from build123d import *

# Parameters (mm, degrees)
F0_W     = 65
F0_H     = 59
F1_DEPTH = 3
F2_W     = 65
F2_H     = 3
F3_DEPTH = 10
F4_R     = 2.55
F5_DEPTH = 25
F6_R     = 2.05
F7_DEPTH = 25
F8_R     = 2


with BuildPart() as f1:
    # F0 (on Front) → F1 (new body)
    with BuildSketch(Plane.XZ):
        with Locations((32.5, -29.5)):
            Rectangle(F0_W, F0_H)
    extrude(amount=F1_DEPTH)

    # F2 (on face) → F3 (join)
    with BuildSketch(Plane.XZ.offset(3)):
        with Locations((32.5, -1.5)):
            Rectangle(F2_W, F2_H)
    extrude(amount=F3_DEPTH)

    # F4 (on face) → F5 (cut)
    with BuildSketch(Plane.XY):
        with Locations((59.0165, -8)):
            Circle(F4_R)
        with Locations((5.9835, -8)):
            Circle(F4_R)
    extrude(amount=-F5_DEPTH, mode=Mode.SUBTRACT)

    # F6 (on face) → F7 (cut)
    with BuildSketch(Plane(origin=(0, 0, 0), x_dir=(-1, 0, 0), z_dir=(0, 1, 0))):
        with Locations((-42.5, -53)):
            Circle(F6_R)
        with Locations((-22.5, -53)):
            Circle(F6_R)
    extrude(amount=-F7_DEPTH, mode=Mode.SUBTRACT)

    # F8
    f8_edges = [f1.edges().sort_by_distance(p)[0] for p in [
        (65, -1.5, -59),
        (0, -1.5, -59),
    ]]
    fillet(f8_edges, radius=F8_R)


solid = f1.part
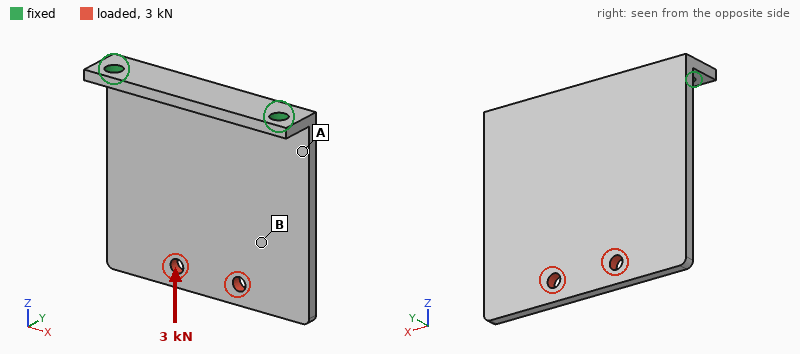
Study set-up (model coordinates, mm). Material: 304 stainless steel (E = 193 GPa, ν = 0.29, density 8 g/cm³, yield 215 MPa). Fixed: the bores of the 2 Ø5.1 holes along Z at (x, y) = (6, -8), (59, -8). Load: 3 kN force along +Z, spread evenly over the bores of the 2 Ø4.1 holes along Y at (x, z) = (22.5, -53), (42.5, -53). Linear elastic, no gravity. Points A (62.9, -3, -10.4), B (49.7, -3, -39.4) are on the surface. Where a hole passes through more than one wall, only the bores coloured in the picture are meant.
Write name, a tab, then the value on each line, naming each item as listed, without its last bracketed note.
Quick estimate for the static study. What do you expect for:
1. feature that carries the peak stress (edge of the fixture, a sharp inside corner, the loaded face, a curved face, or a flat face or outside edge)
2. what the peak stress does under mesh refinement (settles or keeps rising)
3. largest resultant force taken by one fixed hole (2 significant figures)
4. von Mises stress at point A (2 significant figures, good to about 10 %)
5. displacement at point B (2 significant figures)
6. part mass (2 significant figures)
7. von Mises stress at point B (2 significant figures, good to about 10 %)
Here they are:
feature that carries the peak stress	edge of the fixture
what the peak stress does under mesh refinement	keeps rising
largest resultant force taken by one fixed hole	1.5 kN
von Mises stress at point A	39 MPa
displacement at point B	0.10 mm
part mass	110 g
von Mises stress at point B	21 MPa
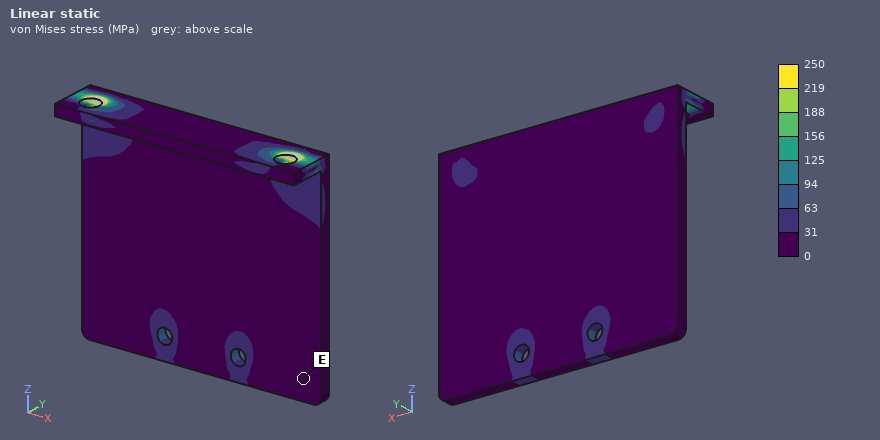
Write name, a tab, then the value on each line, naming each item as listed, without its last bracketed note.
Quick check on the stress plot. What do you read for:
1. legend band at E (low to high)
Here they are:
legend band at E	0 to 31 MPa
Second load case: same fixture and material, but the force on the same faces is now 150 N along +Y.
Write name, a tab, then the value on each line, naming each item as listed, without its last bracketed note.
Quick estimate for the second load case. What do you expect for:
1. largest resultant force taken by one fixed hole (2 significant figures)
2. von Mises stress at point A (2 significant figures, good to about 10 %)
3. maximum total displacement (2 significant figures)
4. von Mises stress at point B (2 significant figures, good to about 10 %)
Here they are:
largest resultant force taken by one fixed hole	78 N
von Mises stress at point A	69 MPa
maximum total displacement	0.43 mm
von Mises stress at point B	24 MPa
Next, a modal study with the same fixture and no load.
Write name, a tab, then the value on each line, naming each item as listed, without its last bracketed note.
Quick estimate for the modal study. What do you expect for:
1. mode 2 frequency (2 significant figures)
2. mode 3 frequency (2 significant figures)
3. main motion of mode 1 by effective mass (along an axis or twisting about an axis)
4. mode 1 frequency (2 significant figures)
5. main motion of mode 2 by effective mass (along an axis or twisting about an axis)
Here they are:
mode 2 frequency	1500 Hz
mode 3 frequency	3800 Hz
main motion of mode 1 by effective mass	along Y
mode 1 frequency	580 Hz
main motion of mode 2 by effective mass	twisting about Z
